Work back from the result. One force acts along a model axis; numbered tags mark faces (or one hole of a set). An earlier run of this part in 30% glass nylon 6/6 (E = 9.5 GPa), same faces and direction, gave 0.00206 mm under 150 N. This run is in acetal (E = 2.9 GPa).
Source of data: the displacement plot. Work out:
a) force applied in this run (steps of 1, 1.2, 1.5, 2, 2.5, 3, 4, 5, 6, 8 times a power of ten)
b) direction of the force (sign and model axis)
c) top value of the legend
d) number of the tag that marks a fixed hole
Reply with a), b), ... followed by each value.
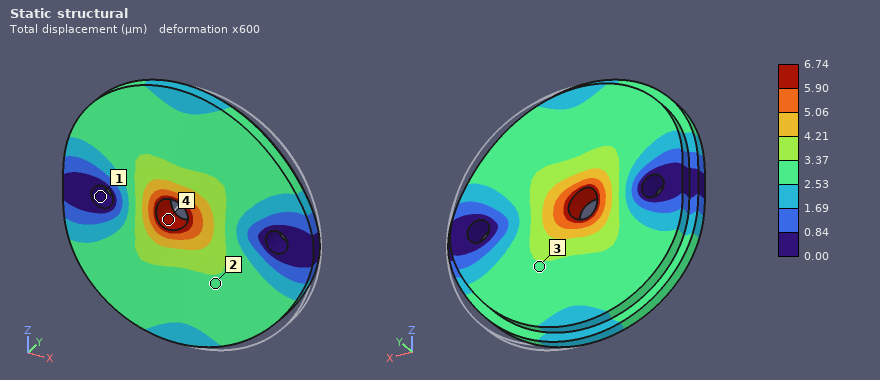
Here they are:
a) 150 N
b) -X
c) 6.74 µm
d) 1
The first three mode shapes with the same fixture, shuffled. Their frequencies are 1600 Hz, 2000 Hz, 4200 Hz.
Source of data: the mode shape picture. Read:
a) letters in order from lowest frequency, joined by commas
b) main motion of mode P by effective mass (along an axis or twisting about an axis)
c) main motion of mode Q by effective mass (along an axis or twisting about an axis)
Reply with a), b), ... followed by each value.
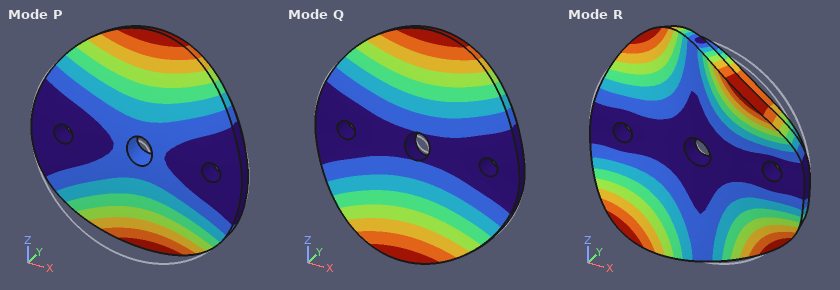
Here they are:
a) Q, P, R
b) along Y
c) twisting about X
